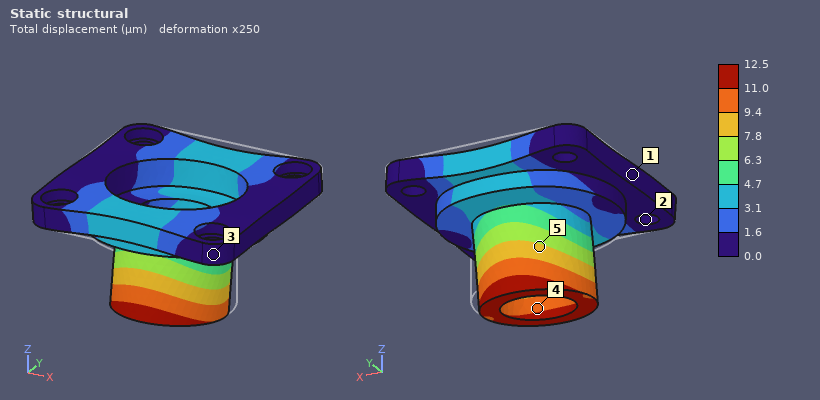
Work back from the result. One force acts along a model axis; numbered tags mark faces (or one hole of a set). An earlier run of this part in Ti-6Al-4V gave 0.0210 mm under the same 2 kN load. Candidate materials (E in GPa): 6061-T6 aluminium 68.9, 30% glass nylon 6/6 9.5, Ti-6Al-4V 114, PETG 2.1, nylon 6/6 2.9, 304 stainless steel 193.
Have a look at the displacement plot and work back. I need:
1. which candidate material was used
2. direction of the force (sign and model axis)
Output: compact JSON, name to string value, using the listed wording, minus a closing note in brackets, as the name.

{"which candidate material was used": "304 stainless steel", "direction of the force": "-Y"}
